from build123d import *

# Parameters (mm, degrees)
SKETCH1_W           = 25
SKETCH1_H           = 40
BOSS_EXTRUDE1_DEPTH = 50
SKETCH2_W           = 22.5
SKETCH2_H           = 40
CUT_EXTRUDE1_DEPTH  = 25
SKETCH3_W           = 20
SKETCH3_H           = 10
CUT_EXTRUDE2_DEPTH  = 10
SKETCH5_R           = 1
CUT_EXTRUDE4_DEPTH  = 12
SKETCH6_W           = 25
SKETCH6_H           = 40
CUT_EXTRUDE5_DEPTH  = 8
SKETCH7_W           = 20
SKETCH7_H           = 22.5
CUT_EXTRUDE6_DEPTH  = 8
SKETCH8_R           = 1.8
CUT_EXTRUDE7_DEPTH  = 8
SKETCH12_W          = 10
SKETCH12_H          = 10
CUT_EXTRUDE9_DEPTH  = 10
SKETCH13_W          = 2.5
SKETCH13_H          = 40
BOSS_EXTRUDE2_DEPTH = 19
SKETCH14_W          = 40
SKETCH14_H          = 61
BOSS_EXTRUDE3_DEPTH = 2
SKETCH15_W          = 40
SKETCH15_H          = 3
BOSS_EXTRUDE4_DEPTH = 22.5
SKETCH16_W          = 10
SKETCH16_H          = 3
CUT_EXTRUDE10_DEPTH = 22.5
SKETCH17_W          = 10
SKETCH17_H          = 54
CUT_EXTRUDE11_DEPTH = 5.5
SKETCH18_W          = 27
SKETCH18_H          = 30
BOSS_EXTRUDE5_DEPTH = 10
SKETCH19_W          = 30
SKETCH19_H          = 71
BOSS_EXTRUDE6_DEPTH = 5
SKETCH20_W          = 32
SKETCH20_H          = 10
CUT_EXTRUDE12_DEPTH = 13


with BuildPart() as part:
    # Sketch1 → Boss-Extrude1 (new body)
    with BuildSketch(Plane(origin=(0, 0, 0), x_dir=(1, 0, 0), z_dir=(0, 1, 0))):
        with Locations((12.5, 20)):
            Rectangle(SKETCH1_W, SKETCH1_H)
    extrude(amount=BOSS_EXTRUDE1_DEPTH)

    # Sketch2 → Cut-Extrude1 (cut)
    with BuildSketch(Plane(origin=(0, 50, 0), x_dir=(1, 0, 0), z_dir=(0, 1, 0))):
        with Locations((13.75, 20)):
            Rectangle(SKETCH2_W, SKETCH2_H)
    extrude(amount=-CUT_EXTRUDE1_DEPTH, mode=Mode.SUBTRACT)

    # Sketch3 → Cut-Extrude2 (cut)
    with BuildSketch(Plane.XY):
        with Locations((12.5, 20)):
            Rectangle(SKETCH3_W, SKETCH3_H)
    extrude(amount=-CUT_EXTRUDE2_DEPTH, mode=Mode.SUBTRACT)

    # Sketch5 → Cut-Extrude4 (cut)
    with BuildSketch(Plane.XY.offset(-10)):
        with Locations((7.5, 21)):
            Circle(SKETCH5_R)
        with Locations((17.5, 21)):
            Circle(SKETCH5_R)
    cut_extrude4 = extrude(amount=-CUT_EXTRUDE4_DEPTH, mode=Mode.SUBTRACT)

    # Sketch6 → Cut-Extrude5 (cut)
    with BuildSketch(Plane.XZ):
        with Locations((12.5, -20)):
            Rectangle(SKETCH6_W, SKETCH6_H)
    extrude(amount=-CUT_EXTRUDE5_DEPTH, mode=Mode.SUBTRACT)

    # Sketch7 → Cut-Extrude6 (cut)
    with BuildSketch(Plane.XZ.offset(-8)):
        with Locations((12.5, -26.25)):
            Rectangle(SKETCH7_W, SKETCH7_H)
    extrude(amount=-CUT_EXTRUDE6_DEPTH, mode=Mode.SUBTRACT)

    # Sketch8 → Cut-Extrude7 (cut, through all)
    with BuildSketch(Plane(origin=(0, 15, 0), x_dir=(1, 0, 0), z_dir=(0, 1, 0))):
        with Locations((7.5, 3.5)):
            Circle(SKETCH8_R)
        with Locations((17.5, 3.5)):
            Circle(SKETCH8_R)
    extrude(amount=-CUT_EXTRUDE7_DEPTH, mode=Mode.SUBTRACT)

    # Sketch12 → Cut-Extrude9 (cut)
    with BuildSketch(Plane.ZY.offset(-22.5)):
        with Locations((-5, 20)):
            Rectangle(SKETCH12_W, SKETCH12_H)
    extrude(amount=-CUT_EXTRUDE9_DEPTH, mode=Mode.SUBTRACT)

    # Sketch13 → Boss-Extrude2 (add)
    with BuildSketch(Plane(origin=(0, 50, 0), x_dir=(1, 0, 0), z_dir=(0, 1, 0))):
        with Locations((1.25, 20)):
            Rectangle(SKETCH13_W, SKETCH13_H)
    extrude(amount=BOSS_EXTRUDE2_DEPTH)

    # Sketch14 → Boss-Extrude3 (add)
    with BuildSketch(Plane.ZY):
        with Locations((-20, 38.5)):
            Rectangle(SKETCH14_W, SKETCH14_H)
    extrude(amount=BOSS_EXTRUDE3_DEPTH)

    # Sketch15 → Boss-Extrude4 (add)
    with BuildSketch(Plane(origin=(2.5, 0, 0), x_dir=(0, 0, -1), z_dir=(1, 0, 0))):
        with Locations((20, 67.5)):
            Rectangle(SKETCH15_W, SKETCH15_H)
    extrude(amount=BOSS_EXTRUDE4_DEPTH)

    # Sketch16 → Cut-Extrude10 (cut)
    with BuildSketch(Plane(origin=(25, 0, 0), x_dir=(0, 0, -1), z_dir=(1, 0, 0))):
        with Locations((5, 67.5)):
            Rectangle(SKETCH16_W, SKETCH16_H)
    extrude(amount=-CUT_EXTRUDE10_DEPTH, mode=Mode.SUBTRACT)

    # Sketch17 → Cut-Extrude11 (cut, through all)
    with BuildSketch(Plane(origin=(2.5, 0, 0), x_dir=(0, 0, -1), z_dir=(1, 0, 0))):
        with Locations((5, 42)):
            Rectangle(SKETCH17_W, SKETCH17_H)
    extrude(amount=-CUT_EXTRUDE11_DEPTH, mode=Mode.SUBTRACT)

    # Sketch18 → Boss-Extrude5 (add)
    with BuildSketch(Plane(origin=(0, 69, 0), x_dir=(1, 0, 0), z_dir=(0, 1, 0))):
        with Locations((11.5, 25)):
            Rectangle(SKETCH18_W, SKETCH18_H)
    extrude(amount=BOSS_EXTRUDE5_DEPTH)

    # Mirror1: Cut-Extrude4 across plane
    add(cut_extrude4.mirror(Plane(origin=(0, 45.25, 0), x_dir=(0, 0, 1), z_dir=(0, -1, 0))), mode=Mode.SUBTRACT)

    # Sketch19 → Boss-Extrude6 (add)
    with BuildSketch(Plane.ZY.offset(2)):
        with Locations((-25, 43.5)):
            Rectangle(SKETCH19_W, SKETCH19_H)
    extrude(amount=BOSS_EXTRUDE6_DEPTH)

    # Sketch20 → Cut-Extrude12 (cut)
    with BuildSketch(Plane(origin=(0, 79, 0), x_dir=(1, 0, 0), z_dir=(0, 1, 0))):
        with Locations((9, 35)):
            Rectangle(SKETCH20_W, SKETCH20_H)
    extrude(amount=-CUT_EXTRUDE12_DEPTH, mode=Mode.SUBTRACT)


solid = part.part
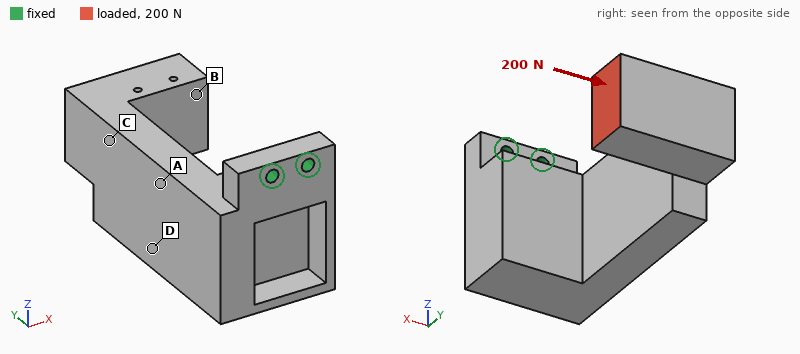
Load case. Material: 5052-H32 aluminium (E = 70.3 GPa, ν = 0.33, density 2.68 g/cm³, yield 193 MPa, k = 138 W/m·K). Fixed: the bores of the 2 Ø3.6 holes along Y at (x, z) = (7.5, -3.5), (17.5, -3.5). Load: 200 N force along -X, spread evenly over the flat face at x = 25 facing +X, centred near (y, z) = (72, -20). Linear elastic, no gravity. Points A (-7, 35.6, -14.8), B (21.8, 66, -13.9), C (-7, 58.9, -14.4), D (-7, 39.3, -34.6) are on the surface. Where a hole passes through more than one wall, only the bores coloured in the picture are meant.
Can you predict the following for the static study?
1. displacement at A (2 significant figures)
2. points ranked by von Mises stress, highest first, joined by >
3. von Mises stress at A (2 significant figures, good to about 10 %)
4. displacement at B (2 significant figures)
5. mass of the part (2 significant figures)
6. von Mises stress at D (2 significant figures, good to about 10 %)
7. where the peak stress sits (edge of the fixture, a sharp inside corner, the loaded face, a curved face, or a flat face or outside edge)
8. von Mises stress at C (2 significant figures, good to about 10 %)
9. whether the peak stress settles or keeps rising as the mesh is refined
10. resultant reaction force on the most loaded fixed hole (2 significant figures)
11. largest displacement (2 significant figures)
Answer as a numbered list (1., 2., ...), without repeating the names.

1. 0.046 mm
2. A > D > C > B
3. 17 MPa
4. 0.14 mm
5. 92 g
6. 14 MPa
7. edge of the fixture
8. 6.9 MPa
9. keeps rising
10. 700 N
11. 0.18 mm
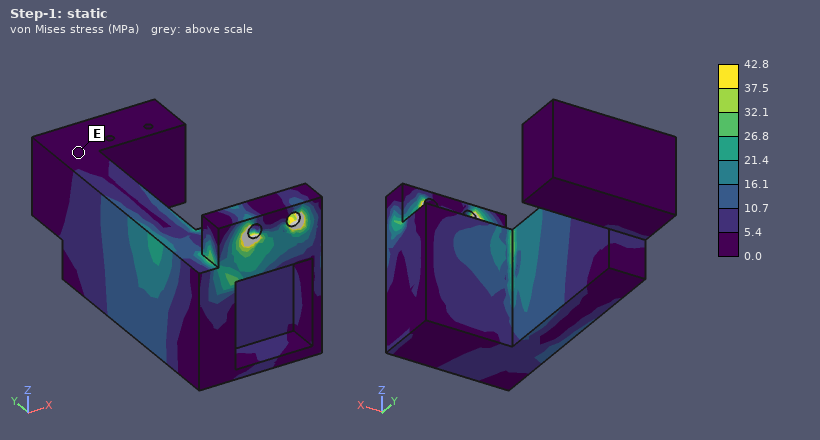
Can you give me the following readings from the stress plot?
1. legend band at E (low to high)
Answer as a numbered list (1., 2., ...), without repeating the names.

1. 0.0 to 5.4 MPa
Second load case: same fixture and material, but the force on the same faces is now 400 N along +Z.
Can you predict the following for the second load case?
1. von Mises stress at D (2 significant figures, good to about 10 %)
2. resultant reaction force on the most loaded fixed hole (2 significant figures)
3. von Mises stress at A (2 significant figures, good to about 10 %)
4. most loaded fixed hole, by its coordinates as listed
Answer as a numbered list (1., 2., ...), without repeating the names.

1. 19 MPa
2. 680 N
3. 20 MPa
4. (17.5, -3.5)
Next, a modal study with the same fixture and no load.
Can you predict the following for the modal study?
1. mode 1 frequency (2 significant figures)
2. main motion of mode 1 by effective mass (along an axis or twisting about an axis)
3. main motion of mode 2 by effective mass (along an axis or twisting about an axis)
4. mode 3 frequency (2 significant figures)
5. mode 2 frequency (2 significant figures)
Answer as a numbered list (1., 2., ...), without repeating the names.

1. 790 Hz
2. along Z
3. along X
4. 3500 Hz
5. 1100 Hz
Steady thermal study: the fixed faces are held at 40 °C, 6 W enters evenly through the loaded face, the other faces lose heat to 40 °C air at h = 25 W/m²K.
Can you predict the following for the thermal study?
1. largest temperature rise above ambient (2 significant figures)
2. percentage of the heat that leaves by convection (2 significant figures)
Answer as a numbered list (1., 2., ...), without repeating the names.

1. 14 K
2. 26 %
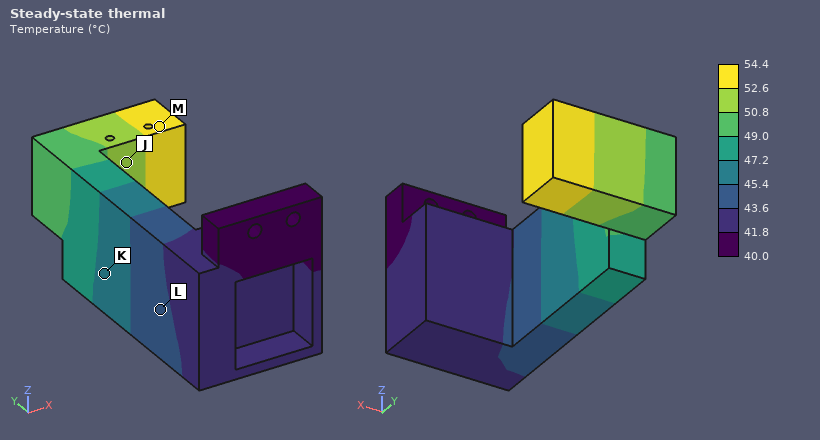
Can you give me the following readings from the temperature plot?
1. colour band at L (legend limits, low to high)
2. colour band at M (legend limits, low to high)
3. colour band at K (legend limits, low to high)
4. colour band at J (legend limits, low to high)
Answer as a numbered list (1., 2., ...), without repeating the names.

1. 43.6 to 45.4 °C
2. 52.6 to 54.4 °C
3. 45.4 to 47.2 °C
4. 50.8 to 52.6 °C
